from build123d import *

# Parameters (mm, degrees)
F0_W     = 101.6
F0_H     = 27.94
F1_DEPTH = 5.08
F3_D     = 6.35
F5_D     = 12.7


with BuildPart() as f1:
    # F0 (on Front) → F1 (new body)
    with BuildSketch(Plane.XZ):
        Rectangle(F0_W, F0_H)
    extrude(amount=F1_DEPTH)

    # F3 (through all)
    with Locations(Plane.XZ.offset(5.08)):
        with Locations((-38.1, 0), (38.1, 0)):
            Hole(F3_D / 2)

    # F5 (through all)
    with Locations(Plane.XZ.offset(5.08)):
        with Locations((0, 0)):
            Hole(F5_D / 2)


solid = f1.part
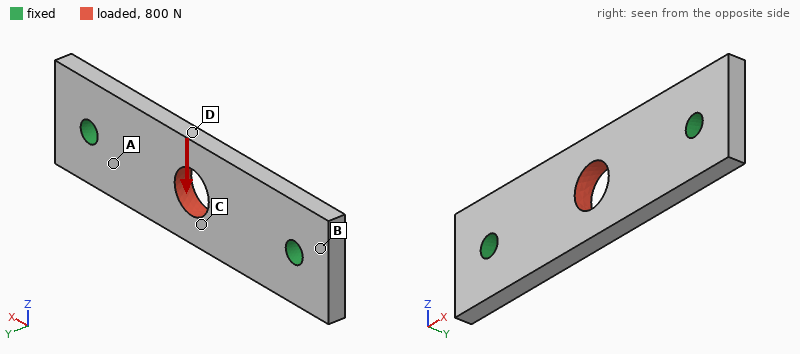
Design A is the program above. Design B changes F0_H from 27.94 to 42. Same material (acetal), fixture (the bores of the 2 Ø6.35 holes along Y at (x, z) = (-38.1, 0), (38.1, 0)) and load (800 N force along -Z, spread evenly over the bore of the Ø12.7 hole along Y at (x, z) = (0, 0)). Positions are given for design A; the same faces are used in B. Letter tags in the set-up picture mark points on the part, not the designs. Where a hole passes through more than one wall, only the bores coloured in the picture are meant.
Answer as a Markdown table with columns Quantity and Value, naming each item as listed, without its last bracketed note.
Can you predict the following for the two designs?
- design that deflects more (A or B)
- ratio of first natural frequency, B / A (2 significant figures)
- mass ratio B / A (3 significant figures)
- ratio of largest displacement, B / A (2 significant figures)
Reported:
| Quantity | Value |
|---|---|
| design that deflects more | A |
| ratio of first natural frequency, B / A | 0.89 |
| mass ratio B / A | 1.54 |
| ratio of largest displacement, B / A | 0.53 |
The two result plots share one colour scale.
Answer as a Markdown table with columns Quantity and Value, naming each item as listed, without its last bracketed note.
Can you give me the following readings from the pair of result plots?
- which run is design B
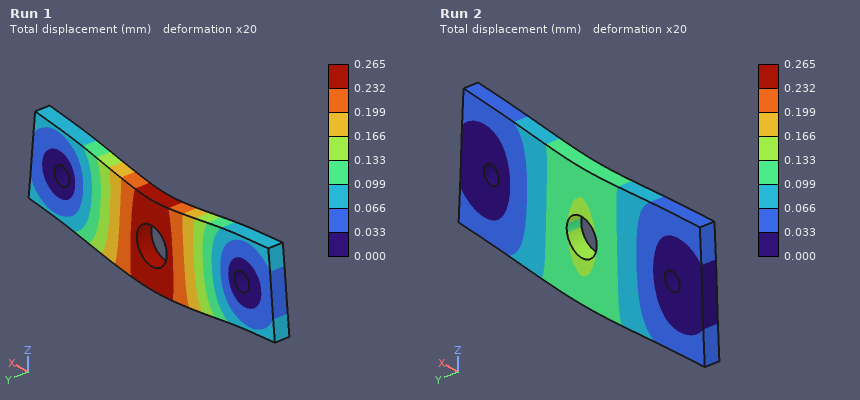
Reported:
| Quantity | Value |
|---|---|
| which run is design B | Run 2 |
